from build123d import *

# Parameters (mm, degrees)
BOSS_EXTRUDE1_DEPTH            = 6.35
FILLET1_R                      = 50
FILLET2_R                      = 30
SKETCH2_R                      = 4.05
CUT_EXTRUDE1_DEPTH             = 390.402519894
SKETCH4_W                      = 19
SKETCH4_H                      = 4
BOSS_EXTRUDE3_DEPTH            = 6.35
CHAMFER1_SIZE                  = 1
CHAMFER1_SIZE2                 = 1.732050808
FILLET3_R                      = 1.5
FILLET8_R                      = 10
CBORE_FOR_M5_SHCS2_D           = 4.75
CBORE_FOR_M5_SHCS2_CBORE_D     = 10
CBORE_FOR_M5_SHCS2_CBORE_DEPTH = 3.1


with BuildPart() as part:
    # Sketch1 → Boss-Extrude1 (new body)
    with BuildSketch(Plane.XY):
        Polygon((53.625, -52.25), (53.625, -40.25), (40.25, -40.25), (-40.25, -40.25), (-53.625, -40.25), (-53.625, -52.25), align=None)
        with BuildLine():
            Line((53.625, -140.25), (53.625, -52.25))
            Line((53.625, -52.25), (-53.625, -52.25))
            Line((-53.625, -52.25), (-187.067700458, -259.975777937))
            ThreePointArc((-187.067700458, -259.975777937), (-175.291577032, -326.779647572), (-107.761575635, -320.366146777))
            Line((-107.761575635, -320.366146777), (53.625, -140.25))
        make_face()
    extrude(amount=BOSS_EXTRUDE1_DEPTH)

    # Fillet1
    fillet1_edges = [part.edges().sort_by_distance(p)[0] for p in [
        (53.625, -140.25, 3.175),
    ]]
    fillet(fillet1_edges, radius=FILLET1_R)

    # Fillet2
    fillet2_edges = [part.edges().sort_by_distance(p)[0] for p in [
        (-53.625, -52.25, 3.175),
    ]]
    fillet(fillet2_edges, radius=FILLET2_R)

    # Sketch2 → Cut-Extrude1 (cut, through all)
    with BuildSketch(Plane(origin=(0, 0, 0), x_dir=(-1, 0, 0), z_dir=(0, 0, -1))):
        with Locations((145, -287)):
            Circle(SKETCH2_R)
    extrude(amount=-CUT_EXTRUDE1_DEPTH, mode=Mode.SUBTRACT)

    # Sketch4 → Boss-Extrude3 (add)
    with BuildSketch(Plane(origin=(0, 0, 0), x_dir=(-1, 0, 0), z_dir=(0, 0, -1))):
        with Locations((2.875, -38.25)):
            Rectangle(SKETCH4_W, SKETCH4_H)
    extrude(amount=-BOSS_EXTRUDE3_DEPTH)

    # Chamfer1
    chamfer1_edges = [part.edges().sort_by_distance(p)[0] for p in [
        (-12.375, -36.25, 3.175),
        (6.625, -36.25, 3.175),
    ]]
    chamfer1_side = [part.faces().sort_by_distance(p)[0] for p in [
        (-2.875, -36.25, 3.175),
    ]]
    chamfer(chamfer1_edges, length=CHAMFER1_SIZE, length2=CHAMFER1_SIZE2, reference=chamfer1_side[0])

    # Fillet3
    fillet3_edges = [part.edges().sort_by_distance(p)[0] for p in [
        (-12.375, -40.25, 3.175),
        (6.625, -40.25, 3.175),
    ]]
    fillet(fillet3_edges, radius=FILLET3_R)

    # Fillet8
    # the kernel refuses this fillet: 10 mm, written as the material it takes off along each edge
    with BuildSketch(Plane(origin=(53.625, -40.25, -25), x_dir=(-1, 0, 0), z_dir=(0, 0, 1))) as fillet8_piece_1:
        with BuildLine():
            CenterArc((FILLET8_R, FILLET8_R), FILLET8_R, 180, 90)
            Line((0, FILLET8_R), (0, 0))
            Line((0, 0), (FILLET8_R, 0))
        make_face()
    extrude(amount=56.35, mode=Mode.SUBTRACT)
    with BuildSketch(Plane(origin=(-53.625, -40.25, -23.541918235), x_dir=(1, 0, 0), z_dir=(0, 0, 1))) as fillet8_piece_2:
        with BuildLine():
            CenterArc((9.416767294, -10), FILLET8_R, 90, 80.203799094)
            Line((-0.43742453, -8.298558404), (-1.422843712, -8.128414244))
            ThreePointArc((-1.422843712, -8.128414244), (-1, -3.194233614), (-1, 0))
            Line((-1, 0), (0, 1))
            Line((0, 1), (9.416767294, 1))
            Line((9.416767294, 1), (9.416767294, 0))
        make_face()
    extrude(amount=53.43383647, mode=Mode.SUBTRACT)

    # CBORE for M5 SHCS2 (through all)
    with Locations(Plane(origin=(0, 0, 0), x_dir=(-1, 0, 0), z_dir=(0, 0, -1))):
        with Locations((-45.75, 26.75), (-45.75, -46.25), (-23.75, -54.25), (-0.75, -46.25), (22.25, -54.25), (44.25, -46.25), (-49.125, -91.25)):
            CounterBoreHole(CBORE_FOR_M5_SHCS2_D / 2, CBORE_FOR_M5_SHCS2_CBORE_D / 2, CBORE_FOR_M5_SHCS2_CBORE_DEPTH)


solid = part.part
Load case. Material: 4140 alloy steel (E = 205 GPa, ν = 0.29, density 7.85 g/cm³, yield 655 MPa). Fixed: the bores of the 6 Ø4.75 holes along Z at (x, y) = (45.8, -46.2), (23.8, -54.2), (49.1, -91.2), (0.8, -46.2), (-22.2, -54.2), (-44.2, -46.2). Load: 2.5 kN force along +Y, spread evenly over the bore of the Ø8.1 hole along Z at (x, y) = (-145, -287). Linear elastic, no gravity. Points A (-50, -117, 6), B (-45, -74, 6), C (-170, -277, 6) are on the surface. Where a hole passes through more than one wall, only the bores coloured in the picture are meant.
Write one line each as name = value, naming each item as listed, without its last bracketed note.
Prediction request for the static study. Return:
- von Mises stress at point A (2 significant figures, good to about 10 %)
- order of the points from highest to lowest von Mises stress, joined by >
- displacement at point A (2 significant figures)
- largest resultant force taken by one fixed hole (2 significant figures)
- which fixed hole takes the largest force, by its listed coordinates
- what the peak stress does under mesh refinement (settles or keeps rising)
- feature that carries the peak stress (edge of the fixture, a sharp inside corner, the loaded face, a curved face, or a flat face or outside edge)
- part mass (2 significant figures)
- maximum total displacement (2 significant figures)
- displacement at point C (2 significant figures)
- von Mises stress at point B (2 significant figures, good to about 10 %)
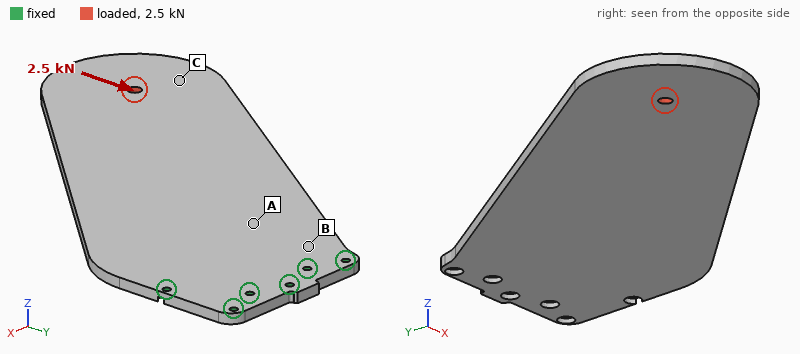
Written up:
von Mises stress at point A = 11 MPa
order of the points from highest to lowest von Mises stress, joined by > = B > A > C
displacement at point A = 15 µm
largest resultant force taken by one fixed hole = 3.0 kN
which fixed hole takes the largest force, by its listed coordinates = (-44.2, -46.2)
what the peak stress does under mesh refinement = keeps rising
feature that carries the peak stress = edge of the fixture
part mass = 1.9 kg
maximum total displacement = 85 µm
displacement at point C = 73 µm
von Mises stress at point B = 21 MPa
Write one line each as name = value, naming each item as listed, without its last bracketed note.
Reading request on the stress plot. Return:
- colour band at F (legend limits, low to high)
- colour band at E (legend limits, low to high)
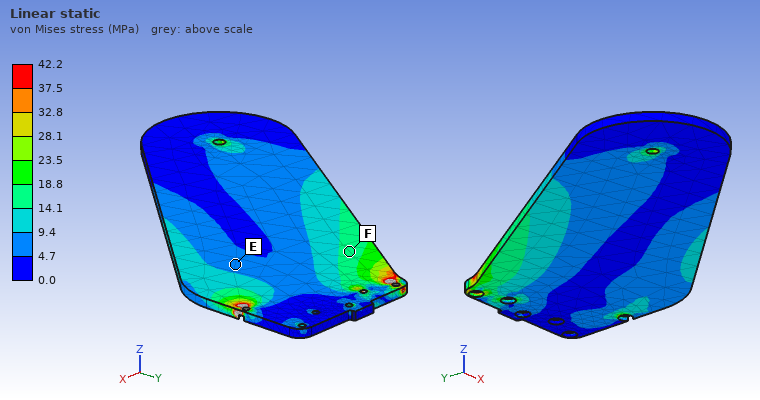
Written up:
colour band at F = 14.1 to 18.8 MPa
colour band at E = 4.7 to 9.4 MPa
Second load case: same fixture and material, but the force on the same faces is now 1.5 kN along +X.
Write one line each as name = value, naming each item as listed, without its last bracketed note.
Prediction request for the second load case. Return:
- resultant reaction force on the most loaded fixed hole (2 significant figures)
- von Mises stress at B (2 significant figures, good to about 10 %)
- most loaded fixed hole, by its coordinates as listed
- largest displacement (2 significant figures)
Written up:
resultant reaction force on the most loaded fixed hole = 2.9 kN
von Mises stress at B = 15 MPa
most loaded fixed hole, by its coordinates as listed = (49.1, -91.2)
largest displacement = 64 µm
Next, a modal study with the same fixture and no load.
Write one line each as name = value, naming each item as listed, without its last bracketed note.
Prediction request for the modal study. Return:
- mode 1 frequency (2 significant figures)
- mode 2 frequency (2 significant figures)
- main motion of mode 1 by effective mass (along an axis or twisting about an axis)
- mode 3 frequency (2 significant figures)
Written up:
mode 1 frequency = 58 Hz
mode 2 frequency = 320 Hz
main motion of mode 1 by effective mass = along Z
mode 3 frequency = 370 Hz
